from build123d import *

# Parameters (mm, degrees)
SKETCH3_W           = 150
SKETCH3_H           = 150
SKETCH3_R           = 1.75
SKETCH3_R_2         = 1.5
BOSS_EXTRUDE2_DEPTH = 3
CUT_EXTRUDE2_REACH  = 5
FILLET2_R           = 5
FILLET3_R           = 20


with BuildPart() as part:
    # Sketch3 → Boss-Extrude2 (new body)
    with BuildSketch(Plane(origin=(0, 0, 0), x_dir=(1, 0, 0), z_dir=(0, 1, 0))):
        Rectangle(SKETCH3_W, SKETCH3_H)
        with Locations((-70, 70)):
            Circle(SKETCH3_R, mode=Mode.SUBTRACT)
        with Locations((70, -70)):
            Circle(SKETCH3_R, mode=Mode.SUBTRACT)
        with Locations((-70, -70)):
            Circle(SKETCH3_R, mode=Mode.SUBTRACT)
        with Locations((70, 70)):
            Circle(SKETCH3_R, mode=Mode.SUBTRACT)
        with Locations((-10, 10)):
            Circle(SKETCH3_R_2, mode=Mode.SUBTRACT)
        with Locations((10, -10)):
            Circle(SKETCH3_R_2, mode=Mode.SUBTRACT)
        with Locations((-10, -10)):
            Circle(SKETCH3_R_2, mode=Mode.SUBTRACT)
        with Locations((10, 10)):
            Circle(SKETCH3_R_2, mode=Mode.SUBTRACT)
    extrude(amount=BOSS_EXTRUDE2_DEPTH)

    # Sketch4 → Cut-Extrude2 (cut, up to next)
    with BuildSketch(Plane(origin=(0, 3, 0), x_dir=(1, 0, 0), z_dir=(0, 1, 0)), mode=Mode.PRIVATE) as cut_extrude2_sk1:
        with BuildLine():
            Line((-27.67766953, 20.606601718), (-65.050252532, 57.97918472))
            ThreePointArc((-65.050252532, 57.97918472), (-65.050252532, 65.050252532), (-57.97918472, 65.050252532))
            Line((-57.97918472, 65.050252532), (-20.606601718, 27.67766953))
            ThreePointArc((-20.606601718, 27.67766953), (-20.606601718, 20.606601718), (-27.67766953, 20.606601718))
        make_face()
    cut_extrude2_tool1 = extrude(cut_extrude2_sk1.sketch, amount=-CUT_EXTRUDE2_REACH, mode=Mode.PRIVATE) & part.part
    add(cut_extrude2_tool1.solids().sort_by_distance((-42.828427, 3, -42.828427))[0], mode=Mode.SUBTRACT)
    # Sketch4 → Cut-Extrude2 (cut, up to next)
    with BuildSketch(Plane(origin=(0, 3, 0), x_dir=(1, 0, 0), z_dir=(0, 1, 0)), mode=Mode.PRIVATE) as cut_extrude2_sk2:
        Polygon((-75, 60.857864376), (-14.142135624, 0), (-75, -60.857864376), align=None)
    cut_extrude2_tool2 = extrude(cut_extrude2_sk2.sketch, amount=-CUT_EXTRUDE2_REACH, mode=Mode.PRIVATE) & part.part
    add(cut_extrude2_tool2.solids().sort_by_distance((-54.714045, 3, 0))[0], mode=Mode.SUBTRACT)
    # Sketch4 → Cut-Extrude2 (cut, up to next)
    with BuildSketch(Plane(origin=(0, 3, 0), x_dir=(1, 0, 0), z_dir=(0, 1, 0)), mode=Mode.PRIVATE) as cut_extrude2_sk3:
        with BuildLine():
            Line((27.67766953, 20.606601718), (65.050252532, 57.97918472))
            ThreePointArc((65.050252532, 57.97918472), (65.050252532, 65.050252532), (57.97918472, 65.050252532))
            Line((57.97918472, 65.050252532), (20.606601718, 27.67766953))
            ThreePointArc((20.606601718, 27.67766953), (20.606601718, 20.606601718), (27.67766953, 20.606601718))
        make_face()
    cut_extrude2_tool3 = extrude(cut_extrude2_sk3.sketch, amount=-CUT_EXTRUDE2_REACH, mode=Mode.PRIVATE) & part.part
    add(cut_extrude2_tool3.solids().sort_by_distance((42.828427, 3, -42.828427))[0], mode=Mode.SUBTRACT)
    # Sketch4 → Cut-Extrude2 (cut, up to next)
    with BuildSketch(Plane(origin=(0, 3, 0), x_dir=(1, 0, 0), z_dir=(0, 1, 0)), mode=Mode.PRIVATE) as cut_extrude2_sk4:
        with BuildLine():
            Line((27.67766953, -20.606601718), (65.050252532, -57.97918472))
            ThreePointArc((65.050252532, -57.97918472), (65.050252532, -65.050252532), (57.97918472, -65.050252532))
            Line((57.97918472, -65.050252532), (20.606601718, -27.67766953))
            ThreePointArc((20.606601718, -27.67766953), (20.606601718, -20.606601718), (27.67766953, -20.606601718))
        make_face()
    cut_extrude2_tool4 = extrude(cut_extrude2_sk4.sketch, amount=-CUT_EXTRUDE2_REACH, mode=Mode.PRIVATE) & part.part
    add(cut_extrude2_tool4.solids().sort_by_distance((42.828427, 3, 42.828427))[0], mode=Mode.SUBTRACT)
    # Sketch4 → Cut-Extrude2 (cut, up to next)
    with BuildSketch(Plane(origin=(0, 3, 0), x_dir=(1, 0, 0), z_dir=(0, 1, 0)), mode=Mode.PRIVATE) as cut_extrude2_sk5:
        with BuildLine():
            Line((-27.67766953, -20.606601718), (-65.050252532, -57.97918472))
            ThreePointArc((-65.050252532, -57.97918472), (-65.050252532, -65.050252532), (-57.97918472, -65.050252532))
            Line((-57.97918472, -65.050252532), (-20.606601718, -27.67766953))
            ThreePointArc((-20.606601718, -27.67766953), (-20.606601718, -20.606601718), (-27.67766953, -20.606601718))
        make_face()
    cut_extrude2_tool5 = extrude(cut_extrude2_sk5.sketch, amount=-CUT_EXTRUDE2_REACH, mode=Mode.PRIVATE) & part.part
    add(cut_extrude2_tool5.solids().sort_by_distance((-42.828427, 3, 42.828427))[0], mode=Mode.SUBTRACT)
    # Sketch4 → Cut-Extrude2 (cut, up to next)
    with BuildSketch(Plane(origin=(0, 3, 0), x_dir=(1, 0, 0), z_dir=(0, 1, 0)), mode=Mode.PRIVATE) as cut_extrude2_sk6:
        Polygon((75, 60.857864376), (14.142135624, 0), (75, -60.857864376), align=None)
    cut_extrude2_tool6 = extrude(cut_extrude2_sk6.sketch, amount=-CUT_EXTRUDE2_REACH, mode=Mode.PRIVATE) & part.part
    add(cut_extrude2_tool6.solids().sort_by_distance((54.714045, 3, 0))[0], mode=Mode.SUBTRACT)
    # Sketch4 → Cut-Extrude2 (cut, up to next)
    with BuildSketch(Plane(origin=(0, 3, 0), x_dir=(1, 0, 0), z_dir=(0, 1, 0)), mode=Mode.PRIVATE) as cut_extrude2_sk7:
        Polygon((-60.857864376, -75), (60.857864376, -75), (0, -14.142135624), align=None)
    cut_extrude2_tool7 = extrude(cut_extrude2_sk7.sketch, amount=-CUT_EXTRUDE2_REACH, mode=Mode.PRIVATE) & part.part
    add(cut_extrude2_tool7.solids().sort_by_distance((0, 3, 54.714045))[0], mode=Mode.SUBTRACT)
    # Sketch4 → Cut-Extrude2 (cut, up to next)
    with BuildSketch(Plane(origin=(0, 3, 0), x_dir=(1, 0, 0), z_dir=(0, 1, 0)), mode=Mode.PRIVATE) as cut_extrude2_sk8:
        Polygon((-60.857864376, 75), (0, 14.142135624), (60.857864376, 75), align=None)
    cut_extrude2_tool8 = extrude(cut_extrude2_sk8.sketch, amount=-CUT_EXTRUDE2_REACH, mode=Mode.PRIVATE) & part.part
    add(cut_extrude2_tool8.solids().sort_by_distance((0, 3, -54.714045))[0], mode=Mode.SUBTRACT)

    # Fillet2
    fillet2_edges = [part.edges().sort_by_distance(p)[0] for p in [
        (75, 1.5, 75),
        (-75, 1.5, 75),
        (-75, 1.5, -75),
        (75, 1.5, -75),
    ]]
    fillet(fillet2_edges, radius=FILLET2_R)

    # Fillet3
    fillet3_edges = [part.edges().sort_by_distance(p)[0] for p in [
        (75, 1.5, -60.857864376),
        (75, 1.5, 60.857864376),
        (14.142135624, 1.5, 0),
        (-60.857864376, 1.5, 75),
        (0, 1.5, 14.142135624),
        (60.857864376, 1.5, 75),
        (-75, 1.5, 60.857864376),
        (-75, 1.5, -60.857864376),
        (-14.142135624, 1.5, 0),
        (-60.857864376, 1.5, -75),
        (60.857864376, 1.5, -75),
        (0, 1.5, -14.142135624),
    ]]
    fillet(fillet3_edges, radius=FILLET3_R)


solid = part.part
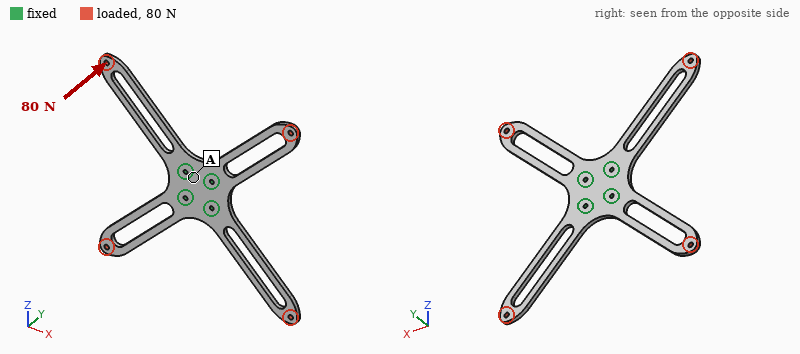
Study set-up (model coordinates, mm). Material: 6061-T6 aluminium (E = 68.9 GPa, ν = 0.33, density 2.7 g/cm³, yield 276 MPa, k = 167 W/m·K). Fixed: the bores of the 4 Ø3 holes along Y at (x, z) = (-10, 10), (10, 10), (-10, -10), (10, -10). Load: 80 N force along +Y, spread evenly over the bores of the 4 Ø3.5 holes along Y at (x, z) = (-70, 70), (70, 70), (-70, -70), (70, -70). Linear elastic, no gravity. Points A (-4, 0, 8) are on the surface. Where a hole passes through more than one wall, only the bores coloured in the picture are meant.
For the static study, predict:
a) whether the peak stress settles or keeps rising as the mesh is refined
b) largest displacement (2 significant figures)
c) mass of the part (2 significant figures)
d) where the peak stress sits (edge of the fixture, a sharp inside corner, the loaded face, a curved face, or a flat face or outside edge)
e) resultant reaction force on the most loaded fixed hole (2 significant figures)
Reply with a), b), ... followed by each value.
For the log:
a) keeps rising
b) 2.1 mm
c) 44 g
d) edge of the fixture
e) 20 N
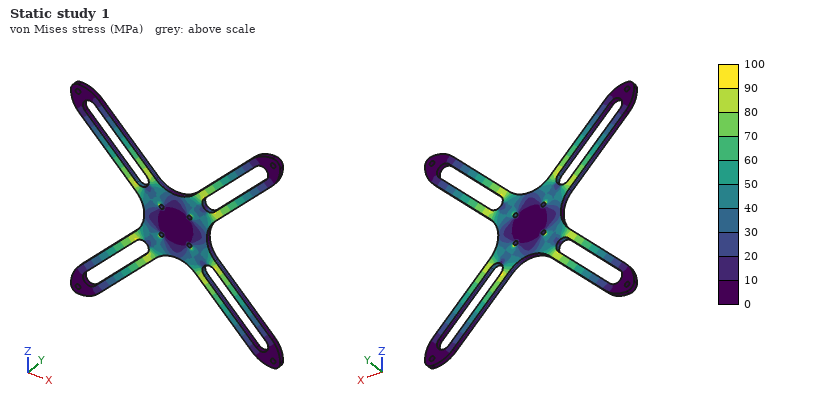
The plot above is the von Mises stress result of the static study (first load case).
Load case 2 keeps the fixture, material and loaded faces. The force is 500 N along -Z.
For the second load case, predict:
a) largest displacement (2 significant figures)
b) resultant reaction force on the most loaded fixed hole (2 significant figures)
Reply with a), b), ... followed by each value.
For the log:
a) 0.56 mm
b) 130 N
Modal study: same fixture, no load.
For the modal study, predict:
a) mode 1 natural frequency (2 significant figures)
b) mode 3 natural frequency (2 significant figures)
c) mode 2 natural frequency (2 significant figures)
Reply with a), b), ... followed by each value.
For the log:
a) 340 Hz
b) 340 Hz
c) 340 Hz
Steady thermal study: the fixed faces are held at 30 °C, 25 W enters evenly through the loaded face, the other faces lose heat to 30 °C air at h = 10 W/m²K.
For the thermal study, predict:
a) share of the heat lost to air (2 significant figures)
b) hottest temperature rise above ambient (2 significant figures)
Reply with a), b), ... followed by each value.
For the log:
a) 19 %
b) 84 K
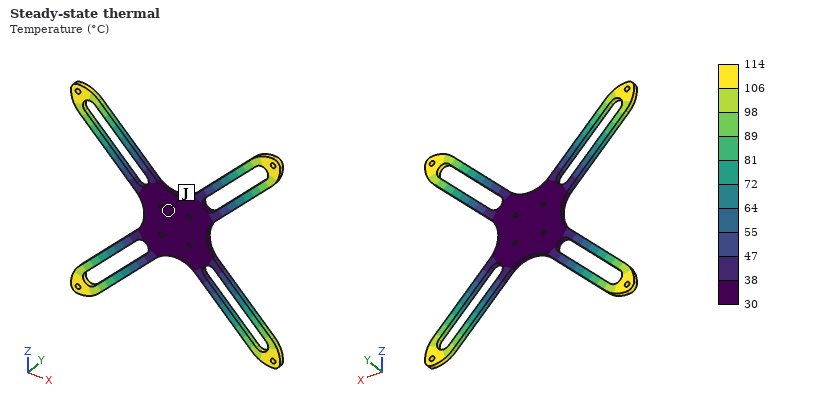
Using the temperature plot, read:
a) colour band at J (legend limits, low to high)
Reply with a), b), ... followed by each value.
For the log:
a) 30 to 38 °C
